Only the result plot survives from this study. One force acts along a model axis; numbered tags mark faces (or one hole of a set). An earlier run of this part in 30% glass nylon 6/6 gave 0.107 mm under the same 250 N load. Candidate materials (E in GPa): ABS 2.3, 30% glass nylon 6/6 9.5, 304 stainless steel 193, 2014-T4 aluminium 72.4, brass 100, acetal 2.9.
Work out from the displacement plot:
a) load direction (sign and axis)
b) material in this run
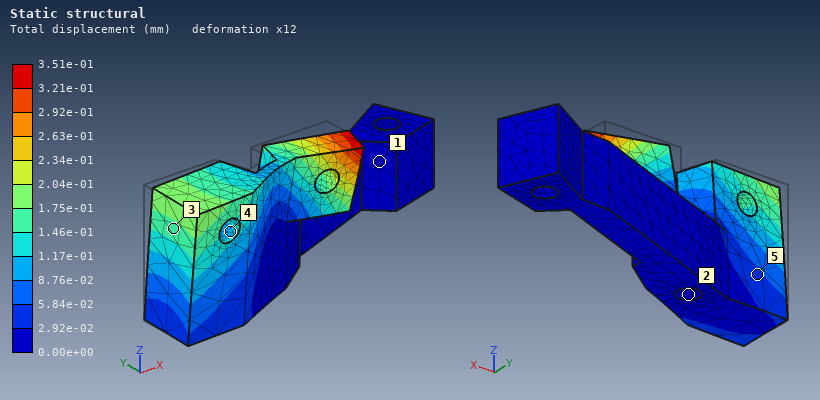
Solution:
-Y
acetal
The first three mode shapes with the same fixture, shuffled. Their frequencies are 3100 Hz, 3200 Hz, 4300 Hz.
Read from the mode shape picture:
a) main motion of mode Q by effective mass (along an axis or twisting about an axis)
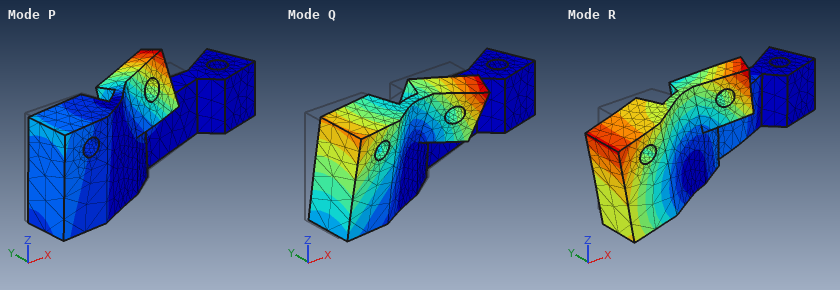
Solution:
along Y
